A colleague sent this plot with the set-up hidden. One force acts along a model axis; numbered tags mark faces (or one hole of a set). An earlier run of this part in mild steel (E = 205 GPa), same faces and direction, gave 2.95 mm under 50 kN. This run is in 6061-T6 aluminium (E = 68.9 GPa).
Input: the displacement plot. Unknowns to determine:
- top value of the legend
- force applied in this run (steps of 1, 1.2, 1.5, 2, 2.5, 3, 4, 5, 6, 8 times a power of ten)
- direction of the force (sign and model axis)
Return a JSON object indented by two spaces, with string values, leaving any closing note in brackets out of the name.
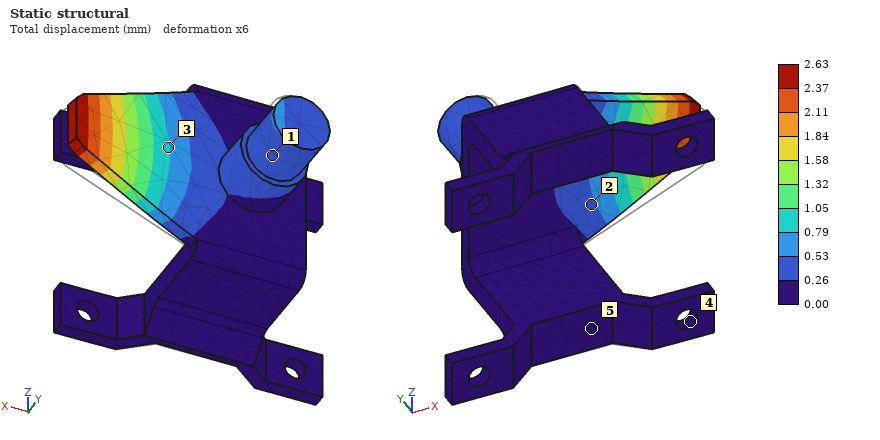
{
  "top value of the legend": "2.63 mm",
  "force applied in this run": "15 kN",
  "direction of the force": "+Y"
}
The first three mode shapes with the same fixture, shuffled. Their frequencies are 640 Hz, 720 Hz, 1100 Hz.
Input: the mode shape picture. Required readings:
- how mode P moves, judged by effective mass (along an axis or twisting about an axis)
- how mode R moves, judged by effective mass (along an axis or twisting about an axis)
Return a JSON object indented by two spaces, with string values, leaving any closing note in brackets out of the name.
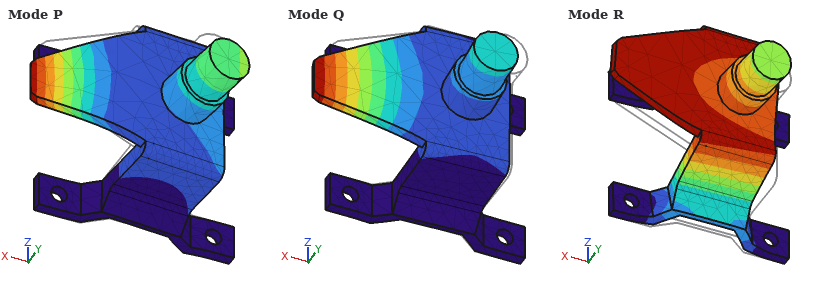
{
  "how mode P moves, judged by effective mass": "along X",
  "how mode R moves, judged by effective mass": "along Z"
}
